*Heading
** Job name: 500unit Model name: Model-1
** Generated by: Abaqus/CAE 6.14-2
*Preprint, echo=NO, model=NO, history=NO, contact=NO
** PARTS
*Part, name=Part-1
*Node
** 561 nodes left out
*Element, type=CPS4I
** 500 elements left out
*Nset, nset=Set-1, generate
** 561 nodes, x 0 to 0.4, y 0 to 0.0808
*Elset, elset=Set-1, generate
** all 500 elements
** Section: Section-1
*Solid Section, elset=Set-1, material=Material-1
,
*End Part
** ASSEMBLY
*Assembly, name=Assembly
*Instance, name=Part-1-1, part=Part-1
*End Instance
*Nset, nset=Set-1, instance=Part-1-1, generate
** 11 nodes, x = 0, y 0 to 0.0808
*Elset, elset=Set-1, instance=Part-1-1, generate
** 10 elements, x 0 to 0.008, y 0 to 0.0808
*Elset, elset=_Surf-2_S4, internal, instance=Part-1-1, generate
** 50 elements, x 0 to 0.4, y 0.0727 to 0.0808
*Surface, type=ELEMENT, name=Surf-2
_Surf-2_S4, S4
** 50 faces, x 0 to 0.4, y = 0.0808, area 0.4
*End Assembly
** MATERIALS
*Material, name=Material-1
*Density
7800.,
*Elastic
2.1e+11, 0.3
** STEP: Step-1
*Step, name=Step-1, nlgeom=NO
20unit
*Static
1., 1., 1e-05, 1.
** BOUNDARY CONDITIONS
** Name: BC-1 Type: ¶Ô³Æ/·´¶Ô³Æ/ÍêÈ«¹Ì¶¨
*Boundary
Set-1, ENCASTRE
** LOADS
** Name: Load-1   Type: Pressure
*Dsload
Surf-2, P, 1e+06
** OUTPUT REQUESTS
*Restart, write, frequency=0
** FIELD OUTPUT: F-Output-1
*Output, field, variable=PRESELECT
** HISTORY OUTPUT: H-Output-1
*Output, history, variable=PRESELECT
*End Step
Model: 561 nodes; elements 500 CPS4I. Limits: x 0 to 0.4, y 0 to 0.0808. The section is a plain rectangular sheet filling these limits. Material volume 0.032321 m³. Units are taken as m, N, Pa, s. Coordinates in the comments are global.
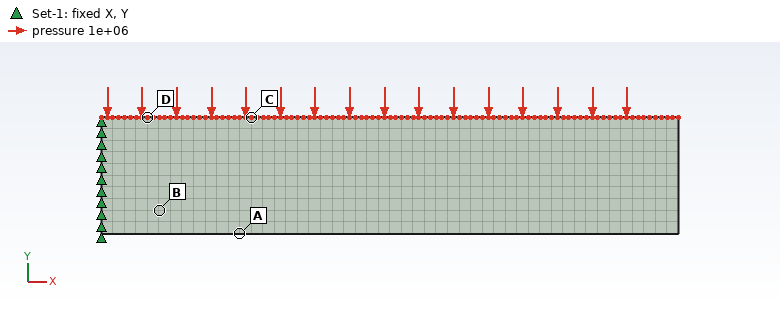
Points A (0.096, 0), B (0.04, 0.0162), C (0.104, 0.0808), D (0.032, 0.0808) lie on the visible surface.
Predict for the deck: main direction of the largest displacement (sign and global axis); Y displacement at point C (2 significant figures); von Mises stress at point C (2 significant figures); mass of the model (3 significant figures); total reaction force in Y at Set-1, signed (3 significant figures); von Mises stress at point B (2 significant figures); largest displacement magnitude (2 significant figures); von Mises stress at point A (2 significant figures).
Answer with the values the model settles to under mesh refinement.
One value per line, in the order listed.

-Y
-4.3e-05 m
3.6e+07 Pa
252 kg
4.00e+05 N
3.3e+07 Pa
3.3e-04 m
3.8e+07 Pa
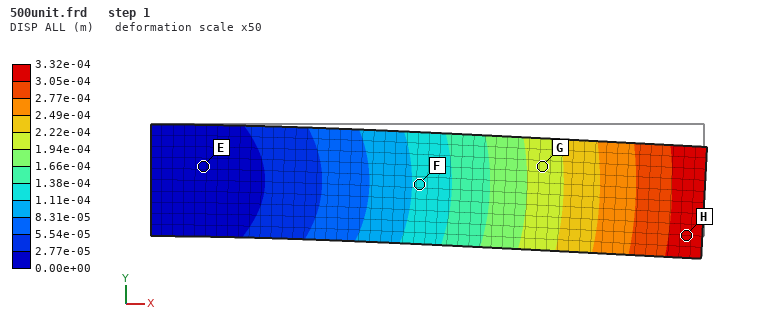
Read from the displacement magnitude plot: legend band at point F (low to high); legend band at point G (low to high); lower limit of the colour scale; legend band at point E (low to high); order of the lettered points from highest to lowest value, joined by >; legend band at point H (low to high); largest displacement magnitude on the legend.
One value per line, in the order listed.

1.11e-04 to 1.38e-04 m
1.94e-04 to 2.22e-04 m
0.00e+00 m
0.00e+00 to 2.77e-05 m
H > G > F > E
3.05e-04 to 3.32e-04 m
3.32e-04 m
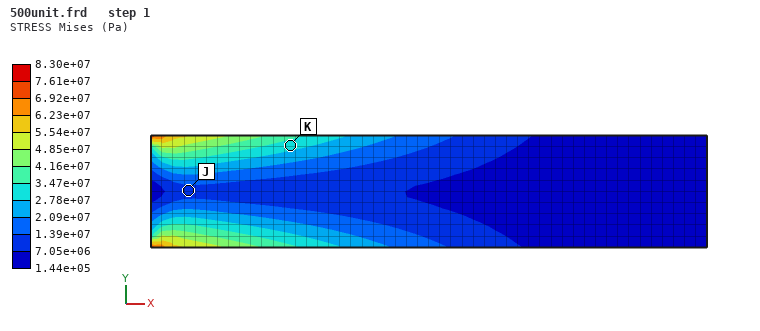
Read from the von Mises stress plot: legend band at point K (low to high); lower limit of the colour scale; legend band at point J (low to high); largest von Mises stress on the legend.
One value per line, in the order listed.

2.78e+07 to 3.47e+07 Pa
1.44e+05 Pa
7.05e+06 to 1.39e+07 Pa
8.30e+07 Pa
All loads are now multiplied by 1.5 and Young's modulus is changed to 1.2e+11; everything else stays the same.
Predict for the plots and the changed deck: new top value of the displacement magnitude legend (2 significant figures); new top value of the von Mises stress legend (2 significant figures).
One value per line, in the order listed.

8.7e-04 m
1.2e+08 Pa
